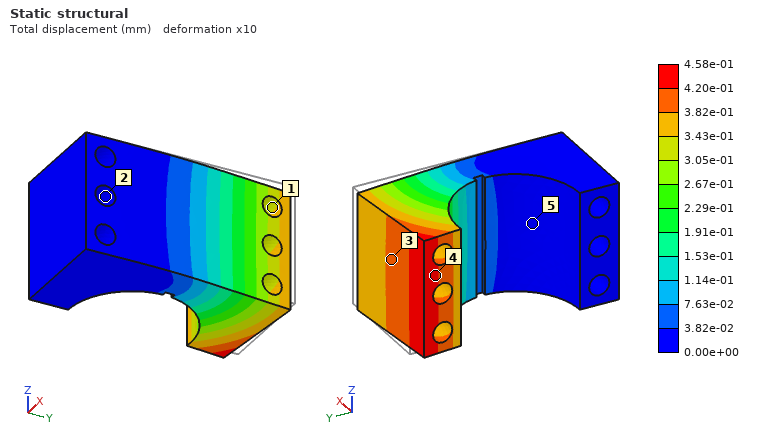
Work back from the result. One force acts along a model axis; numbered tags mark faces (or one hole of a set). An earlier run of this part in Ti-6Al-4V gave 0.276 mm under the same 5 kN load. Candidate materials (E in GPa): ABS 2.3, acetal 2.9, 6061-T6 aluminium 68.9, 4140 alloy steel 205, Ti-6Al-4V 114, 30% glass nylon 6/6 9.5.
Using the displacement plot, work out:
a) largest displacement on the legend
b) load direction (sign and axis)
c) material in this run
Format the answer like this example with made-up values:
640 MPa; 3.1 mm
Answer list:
4.58e-01 mm; -X; 6061-T6 aluminium
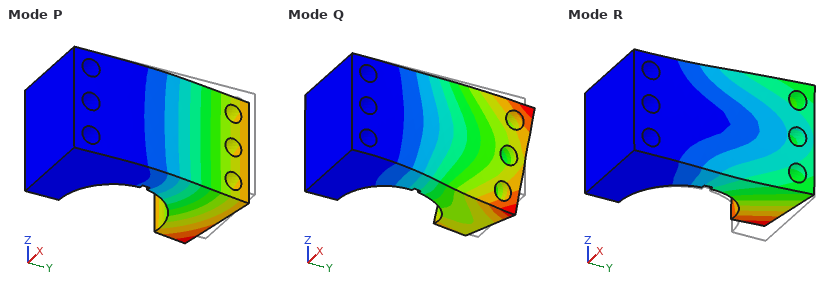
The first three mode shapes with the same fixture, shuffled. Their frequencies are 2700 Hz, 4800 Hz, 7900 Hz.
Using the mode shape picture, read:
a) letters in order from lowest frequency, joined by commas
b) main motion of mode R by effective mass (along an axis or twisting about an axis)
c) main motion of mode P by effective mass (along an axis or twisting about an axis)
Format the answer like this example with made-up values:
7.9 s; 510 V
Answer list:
P, R, Q; along Z; along X
